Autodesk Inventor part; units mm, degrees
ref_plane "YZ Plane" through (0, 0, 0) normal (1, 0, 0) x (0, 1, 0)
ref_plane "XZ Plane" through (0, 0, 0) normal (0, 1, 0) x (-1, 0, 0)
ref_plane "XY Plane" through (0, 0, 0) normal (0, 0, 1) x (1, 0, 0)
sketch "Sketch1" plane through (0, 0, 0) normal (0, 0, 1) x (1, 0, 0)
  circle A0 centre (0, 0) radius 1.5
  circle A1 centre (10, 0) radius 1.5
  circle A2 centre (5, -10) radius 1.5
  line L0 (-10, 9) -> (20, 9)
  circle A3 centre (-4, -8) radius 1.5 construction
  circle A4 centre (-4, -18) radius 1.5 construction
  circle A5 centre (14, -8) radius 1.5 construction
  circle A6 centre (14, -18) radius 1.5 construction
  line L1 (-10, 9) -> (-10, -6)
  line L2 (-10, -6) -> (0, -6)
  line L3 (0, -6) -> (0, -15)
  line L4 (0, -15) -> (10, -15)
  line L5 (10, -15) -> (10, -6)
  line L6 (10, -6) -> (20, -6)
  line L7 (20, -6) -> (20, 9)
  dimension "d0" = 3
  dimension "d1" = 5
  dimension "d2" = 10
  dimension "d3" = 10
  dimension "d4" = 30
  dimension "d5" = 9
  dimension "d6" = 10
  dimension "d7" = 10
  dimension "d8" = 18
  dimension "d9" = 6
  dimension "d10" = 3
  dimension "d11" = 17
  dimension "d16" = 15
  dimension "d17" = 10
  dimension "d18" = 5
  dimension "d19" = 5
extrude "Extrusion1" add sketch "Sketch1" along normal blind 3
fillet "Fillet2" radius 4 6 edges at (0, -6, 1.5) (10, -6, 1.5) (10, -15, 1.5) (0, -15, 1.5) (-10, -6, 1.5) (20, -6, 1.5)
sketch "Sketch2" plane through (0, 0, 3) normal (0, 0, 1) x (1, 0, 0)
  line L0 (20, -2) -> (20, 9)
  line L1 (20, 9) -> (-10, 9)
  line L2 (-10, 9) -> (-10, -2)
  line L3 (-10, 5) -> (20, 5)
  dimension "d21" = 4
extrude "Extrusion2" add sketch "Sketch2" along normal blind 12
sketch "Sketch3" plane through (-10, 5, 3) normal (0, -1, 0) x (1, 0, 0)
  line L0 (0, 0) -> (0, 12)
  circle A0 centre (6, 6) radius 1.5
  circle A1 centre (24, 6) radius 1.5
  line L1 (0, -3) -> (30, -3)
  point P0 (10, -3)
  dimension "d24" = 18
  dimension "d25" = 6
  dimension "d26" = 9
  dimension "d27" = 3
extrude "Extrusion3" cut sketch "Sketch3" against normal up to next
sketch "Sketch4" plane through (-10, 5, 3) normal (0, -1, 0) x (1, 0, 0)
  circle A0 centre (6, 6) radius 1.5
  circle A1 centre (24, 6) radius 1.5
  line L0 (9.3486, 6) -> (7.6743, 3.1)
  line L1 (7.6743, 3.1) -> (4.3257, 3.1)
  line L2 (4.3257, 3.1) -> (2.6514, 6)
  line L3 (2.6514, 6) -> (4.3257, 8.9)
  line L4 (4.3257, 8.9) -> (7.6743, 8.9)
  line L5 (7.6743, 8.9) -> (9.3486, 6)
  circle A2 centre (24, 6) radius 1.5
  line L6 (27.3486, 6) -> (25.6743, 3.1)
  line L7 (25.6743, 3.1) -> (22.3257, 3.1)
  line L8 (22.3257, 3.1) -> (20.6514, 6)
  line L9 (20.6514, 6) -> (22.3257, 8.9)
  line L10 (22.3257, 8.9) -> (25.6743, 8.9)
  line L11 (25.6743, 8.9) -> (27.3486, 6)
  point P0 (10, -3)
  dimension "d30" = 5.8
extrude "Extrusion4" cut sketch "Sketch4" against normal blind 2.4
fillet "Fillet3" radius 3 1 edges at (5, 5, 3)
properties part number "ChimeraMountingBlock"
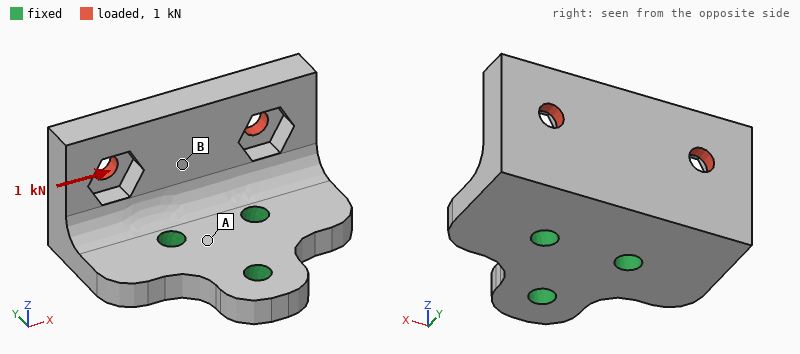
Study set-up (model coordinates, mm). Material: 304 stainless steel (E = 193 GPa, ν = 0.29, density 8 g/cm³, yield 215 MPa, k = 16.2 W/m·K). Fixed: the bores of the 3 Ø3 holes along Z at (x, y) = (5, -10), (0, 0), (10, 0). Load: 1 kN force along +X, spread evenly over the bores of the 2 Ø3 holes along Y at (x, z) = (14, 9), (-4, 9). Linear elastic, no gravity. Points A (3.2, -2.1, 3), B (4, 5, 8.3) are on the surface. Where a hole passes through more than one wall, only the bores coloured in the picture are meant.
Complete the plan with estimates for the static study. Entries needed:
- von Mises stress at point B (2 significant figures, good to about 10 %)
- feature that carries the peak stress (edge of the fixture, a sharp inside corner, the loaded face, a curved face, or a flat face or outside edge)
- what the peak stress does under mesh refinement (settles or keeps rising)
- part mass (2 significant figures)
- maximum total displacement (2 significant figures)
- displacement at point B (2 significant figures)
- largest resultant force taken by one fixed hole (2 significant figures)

28 MPa
edge of the fixture
keeps rising
23 g
14 µm
6.3 µm
950 N
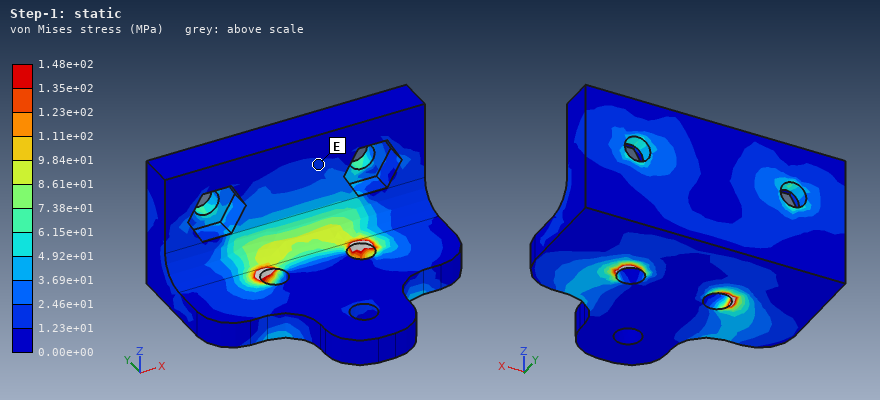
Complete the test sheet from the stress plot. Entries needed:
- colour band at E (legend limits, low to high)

1.23e+01 to 2.46e+01 MPa
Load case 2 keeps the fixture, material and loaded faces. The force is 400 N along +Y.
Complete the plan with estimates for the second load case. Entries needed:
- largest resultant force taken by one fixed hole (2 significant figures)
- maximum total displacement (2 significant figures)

190 N
19 µm
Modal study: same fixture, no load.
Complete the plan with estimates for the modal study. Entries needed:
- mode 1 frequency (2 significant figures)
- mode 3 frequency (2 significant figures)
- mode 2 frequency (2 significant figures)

7700 Hz
19 kHz
11 kHz
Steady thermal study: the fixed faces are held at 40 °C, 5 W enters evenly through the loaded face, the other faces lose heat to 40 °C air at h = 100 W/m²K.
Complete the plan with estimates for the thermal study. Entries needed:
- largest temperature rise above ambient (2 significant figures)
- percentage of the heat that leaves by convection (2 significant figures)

38 K
52 %
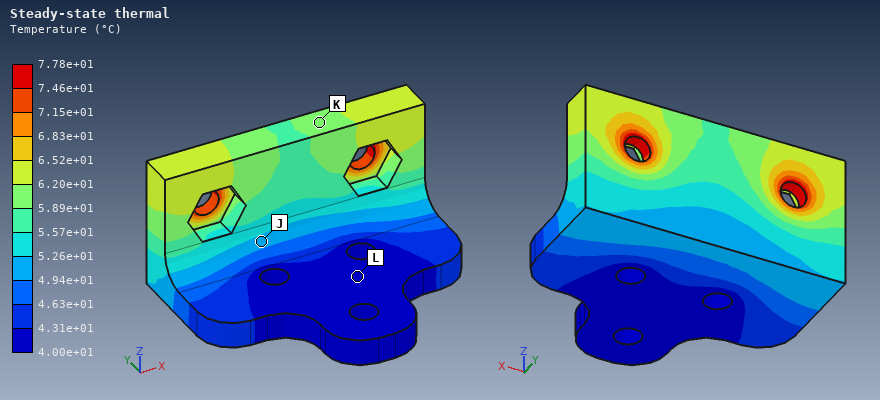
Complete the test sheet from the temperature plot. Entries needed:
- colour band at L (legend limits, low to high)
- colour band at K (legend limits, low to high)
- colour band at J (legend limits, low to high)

4.00e+01 to 4.31e+01 °C
5.89e+01 to 6.20e+01 °C
4.94e+01 to 5.26e+01 °C
